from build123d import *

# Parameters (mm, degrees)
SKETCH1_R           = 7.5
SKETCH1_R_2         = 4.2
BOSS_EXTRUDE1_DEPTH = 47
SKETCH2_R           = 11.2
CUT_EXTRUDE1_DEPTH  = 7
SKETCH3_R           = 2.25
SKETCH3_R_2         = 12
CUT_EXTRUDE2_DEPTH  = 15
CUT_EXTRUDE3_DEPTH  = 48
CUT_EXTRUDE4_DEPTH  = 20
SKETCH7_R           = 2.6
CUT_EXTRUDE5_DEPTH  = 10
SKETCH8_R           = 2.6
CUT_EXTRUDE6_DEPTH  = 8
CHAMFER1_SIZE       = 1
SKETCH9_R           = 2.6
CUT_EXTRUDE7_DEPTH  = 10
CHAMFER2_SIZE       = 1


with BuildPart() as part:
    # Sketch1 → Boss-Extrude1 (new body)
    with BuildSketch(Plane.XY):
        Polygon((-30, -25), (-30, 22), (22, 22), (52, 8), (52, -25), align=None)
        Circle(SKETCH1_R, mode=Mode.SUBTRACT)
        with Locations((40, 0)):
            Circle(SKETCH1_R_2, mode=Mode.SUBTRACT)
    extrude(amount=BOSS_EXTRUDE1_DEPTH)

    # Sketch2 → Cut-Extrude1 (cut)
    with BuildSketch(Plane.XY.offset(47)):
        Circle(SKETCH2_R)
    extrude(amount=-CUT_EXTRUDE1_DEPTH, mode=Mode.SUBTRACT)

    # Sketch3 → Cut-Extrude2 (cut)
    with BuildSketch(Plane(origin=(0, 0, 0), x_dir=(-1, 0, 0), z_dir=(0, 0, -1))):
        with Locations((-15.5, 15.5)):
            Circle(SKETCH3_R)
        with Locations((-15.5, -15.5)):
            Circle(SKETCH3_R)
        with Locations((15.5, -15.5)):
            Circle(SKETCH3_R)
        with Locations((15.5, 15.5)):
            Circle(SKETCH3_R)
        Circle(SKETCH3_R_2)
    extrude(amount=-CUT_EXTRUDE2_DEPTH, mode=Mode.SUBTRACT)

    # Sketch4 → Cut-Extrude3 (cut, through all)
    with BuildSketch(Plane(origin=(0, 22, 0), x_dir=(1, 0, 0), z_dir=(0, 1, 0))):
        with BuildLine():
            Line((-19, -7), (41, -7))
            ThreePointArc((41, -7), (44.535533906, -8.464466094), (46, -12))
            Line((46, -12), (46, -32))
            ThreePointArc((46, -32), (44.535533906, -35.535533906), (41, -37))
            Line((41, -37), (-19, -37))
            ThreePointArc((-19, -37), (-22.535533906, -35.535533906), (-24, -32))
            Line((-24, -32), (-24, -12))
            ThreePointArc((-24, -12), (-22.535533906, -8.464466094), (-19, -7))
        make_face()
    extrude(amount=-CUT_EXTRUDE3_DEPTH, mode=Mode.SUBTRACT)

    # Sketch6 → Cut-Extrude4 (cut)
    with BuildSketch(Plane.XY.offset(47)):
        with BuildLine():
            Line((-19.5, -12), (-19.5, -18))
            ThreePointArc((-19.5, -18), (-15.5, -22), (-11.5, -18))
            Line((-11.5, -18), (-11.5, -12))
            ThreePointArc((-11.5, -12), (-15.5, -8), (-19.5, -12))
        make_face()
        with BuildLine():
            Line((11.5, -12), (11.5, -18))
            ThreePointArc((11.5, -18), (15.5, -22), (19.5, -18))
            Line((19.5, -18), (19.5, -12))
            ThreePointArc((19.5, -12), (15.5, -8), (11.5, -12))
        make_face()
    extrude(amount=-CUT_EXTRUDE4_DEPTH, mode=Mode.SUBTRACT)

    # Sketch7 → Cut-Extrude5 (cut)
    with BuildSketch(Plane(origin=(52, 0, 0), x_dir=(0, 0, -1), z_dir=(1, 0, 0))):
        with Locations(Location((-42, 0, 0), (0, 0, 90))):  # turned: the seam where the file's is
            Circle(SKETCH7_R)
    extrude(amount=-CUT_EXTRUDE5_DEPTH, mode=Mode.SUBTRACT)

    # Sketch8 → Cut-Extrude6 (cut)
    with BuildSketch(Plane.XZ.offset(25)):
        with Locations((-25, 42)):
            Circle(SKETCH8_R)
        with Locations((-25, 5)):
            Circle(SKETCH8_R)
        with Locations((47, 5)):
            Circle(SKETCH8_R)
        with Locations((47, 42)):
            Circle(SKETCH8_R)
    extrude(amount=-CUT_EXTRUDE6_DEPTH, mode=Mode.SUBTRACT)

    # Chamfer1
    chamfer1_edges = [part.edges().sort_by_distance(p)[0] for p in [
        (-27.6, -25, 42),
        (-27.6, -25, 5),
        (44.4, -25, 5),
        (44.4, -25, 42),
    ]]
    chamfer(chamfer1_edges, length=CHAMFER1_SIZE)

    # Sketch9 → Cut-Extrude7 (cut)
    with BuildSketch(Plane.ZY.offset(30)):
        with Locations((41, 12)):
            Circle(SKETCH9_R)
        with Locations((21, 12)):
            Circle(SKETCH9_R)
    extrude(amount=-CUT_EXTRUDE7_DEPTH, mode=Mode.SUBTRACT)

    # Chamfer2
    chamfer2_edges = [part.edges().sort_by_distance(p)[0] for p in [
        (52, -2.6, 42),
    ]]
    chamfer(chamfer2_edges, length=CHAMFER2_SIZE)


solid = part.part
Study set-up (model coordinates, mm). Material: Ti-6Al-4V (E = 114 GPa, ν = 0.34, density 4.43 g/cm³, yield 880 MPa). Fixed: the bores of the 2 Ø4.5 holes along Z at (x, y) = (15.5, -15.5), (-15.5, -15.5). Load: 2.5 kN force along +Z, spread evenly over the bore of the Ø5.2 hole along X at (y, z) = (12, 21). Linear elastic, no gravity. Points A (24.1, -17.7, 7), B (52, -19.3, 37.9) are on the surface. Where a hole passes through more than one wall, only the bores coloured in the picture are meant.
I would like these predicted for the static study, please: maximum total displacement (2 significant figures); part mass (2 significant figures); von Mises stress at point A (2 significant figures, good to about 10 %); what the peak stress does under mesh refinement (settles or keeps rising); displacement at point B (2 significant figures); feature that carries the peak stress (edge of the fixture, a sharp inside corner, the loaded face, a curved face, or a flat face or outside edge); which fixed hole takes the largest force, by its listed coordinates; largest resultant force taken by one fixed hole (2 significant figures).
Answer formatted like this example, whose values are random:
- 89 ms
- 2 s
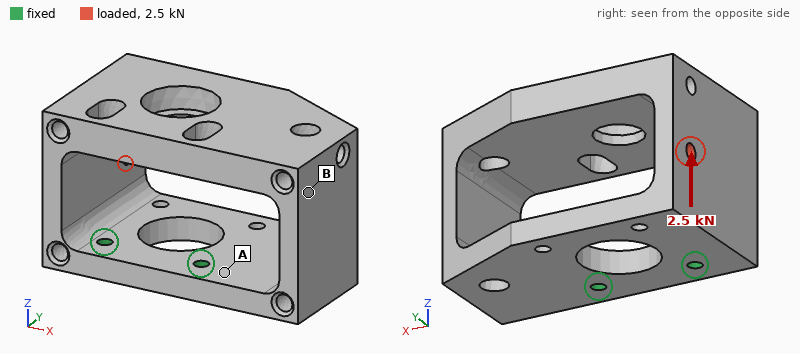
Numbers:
- 0.29 mm
- 290 g
- 64 MPa
- keeps rising
- 0.15 mm
- edge of the fixture
- (-15.5, -15.5)
- 2.7 kN
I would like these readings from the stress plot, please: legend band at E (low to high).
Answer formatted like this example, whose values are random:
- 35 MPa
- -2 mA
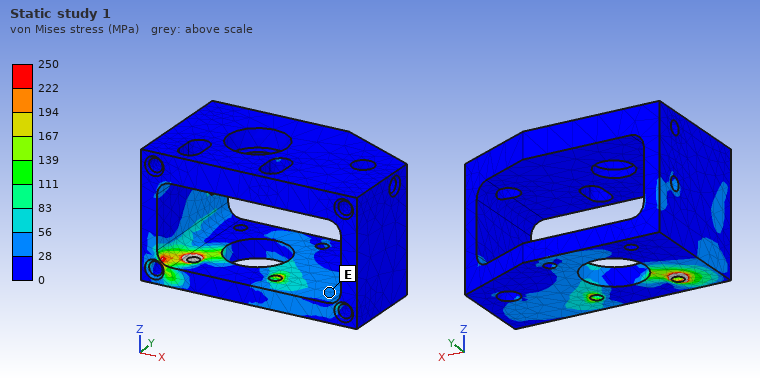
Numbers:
- 28 to 56 MPa
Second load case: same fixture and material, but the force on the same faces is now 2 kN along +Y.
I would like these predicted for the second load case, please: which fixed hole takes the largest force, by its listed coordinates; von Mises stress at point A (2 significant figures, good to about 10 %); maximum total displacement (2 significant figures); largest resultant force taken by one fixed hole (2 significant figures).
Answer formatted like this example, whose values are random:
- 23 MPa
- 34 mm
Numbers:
- (-15.5, -15.5)
- 26 MPa
- 0.15 mm
- 2.5 kN
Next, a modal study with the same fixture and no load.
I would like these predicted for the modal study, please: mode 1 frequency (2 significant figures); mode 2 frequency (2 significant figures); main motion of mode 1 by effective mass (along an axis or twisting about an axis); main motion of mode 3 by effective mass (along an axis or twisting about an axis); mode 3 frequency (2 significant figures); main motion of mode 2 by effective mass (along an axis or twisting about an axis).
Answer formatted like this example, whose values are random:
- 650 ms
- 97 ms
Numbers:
- 1100 Hz
- 1200 Hz
- along Y
- along Z
- 2500 Hz
- along X
